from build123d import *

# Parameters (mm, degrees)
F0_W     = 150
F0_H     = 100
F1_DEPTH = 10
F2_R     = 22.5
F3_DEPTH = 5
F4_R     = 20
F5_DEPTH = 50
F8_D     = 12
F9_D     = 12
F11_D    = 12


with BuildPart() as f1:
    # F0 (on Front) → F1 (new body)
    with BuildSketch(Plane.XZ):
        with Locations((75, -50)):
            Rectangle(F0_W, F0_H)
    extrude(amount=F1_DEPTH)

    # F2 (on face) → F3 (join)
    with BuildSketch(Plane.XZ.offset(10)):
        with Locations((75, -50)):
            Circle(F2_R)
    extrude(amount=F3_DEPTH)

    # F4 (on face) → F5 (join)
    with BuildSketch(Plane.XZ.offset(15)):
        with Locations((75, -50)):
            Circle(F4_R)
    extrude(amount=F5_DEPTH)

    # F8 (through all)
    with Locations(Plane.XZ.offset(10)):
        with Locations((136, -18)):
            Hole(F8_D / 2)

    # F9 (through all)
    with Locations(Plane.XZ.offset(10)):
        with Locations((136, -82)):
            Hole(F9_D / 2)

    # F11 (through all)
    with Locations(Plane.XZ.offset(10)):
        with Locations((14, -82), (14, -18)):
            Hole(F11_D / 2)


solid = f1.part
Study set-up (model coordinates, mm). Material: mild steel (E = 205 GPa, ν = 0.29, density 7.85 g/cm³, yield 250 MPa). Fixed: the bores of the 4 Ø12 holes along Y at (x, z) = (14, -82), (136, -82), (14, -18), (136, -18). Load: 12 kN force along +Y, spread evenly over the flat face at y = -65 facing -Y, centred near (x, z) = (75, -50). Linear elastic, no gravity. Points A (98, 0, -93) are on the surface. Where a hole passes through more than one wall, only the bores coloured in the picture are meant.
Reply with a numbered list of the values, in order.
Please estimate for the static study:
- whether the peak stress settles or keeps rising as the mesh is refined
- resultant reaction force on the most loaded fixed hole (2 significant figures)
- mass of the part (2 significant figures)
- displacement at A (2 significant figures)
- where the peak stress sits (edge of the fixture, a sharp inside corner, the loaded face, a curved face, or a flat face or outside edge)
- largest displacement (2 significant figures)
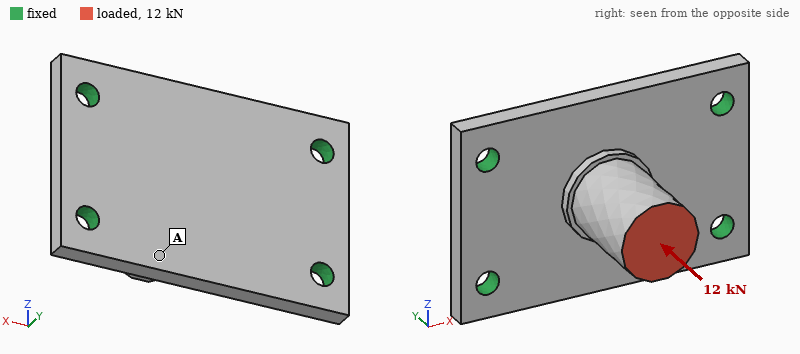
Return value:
1. keeps rising
2. 3.1 kN
3. 1.7 kg
4. 27 µm
5. edge of the fixture
6. 48 µm
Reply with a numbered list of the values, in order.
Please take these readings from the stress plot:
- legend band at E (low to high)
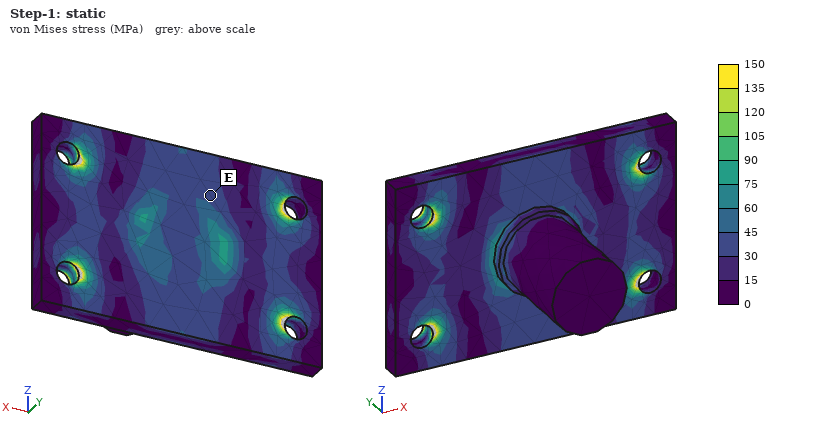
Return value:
1. 30 to 45 MPa
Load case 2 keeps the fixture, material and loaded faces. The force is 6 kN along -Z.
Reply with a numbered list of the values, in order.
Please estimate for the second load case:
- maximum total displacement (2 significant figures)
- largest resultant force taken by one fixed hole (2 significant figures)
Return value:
1. 0.11 mm
2. 3.4 kN
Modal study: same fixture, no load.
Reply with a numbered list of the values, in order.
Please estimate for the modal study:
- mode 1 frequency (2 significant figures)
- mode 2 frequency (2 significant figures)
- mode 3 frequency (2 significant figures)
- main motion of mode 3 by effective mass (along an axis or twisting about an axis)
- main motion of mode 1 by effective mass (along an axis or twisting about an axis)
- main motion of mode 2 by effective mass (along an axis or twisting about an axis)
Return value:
1. 2400 Hz
2. 2600 Hz
3. 3200 Hz
4. along X
5. along Z
6. along Y
